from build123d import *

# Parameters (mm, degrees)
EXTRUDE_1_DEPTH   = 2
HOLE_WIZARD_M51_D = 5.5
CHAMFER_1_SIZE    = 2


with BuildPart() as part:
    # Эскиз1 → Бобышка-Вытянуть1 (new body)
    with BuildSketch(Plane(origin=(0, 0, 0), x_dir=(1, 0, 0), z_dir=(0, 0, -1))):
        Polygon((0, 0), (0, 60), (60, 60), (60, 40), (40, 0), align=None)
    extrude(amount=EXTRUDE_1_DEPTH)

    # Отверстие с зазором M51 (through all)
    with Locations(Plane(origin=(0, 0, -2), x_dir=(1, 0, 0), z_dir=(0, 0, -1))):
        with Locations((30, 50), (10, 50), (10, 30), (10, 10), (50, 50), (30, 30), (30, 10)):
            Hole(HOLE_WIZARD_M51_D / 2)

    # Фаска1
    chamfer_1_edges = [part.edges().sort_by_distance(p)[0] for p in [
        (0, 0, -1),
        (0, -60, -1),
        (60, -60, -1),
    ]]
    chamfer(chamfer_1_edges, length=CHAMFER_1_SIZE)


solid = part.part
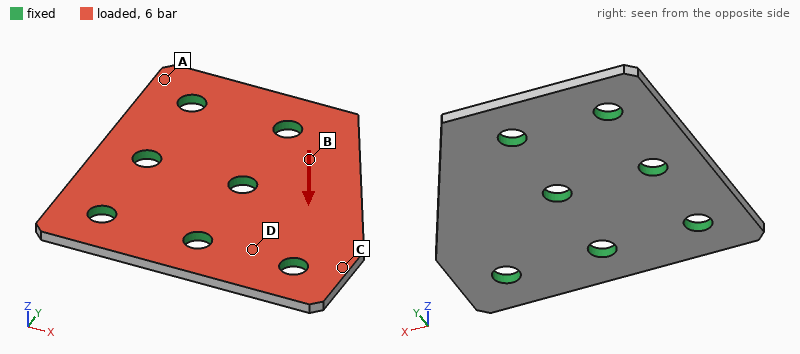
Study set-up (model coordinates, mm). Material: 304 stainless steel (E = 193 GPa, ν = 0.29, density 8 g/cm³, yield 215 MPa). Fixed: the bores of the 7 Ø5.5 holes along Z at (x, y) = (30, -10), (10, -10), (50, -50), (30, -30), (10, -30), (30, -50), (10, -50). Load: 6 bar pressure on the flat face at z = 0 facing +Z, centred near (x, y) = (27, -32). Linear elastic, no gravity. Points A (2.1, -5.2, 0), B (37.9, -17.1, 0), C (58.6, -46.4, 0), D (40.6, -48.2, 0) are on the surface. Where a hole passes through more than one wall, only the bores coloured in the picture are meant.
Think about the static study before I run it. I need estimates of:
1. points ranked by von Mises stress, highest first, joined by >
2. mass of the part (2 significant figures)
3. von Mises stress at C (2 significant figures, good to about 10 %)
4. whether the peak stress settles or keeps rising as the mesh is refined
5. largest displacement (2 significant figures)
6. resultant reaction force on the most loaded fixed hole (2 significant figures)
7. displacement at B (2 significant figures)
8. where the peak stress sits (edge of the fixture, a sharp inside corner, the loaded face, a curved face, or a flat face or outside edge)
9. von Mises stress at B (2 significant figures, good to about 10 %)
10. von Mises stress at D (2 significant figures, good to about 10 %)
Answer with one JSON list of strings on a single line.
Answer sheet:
["C > B > D > A", "48 g", "50 MPa", "keeps rising", "46 µm", "320 N", "11 µm", "edge of the fixture", "36 MPa", "23 MPa"]
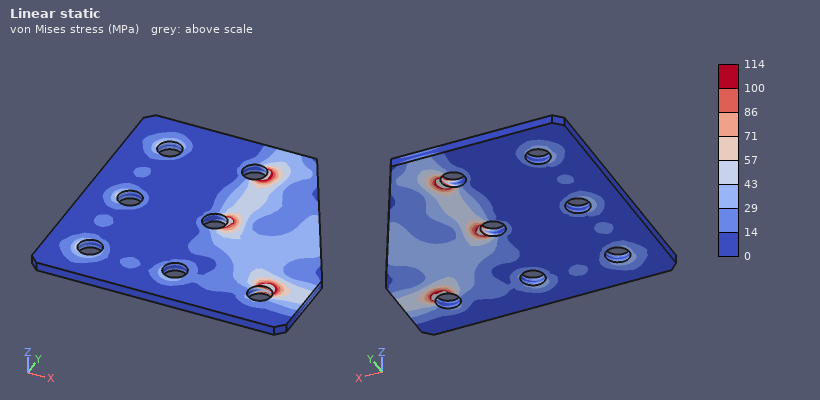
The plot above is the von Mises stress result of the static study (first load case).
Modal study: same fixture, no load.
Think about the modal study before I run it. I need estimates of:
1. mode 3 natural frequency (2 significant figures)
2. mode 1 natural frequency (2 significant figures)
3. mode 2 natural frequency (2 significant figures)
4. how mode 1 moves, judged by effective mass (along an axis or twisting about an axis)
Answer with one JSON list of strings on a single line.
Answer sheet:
["16 kHz", "6200 Hz", "12 kHz", "along Z"]
